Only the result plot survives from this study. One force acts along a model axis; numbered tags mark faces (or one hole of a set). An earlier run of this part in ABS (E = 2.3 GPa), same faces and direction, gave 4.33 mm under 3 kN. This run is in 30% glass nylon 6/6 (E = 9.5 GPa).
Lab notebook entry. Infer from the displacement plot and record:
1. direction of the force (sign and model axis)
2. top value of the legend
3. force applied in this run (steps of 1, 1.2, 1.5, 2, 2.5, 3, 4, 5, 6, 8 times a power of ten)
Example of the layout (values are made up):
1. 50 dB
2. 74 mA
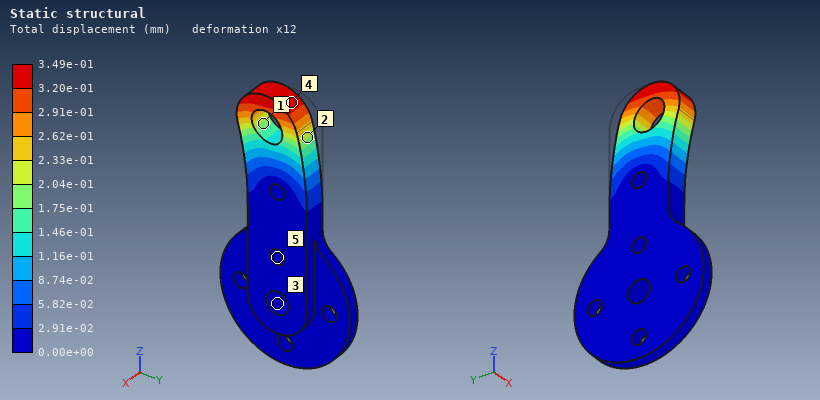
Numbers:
1. -Y
2. 3.49e-01 mm
3. 1 kN
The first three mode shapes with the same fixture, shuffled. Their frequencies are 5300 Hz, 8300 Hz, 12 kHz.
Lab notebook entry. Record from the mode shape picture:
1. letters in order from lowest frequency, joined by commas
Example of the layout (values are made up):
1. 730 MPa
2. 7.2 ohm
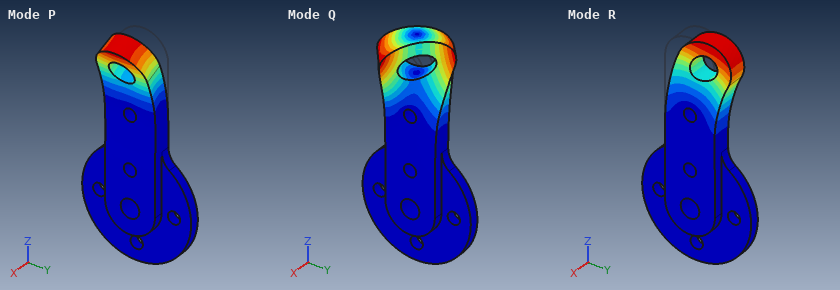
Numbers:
1. P, R, Q
